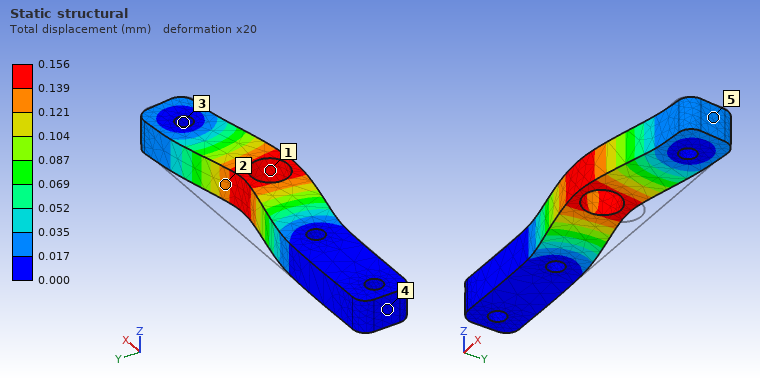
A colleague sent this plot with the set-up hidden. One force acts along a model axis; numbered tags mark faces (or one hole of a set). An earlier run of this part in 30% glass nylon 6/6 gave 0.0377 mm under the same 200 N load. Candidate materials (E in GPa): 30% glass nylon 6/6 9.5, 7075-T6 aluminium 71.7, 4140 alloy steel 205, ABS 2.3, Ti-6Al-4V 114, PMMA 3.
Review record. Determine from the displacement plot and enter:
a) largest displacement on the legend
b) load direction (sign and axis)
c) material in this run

0.156 mm
-Y
ABS
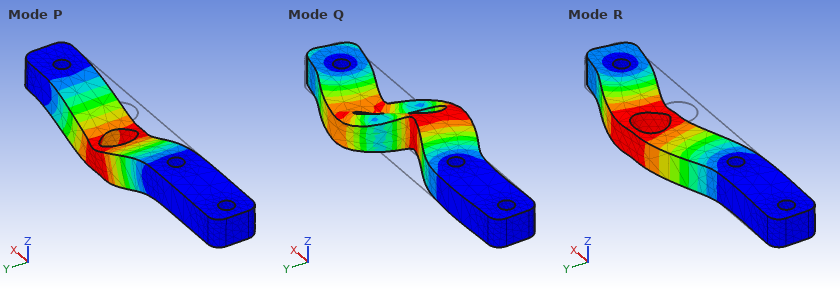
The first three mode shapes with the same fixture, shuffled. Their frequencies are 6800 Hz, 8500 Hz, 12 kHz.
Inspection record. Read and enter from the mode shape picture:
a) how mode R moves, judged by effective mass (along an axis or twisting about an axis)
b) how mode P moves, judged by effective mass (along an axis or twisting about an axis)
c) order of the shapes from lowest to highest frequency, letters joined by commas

along Y
along Z
P, R, Q
